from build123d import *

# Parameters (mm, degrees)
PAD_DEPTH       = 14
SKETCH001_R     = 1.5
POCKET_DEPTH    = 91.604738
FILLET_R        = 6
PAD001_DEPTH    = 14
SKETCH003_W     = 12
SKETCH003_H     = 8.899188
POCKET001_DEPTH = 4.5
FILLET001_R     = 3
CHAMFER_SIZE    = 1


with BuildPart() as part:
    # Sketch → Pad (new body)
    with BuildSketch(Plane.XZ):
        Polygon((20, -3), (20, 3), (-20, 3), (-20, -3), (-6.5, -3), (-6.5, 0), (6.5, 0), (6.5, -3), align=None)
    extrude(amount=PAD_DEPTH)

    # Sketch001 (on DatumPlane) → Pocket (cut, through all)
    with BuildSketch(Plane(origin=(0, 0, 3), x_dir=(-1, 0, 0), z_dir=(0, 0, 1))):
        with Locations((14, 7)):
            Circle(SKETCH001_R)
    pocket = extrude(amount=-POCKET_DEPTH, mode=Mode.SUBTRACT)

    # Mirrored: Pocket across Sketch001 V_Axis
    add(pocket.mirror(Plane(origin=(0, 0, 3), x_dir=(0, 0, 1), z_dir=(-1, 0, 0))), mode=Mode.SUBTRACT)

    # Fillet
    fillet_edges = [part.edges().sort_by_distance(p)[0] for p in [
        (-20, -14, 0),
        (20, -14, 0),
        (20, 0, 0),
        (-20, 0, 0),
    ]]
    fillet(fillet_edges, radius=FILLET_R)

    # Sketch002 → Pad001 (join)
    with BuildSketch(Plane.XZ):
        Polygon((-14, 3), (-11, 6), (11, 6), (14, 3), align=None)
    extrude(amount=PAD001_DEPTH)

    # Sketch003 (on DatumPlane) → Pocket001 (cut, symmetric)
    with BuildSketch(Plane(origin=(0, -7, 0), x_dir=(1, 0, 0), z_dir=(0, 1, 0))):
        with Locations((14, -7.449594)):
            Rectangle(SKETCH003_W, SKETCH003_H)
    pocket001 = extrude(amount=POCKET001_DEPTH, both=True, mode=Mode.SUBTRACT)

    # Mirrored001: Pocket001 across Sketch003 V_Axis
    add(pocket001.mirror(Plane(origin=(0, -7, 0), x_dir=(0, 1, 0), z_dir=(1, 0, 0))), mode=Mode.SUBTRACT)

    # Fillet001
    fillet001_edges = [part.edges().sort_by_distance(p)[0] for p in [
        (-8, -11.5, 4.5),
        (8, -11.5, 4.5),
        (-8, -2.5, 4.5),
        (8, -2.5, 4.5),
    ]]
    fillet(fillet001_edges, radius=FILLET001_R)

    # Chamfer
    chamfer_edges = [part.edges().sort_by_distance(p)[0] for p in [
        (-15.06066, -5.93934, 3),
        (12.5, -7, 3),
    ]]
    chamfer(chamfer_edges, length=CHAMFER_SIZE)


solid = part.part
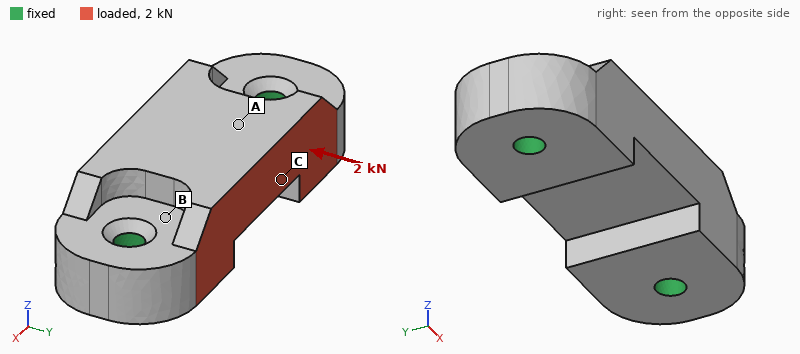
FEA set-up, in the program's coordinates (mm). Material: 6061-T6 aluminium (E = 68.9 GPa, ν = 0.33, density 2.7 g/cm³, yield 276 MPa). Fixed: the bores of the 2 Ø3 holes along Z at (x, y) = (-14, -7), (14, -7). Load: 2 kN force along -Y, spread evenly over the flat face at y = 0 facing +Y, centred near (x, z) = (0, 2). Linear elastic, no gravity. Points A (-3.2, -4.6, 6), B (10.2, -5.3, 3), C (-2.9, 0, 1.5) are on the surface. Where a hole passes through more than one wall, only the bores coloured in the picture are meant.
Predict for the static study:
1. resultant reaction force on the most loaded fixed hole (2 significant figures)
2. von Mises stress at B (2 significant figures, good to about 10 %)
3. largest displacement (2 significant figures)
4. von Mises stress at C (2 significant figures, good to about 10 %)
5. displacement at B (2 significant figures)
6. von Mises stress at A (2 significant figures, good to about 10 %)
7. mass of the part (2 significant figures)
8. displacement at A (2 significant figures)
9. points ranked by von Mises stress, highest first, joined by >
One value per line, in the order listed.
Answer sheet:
1.0 kN
43 MPa
16 µm
25 MPa
5.7 µm
13 MPa
9.1 g
14 µm
B > C > A
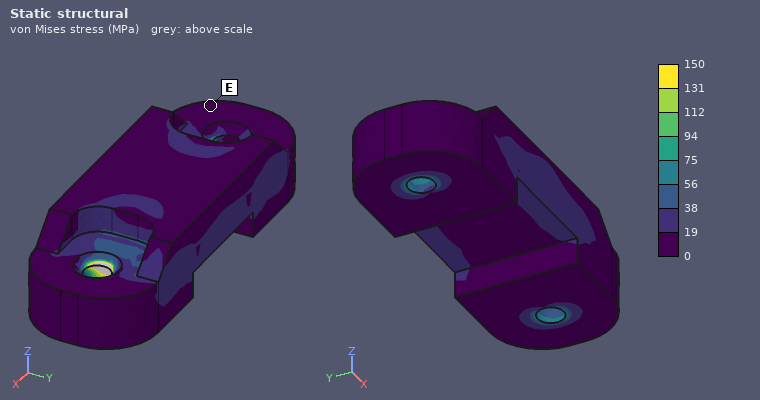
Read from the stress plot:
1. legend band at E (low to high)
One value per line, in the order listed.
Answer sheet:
0 to 19 MPa
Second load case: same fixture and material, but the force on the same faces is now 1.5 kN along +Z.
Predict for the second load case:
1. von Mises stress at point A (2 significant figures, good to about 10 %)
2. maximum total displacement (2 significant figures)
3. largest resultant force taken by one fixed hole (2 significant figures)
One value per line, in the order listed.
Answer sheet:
31 MPa
28 µm
890 N
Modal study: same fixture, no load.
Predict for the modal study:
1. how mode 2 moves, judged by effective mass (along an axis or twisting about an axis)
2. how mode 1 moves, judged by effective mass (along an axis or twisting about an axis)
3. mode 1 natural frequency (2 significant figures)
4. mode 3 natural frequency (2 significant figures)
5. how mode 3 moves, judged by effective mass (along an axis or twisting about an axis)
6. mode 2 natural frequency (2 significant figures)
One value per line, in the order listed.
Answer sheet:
along Z
along Y
24 kHz
41 kHz
along Y
30 kHz
